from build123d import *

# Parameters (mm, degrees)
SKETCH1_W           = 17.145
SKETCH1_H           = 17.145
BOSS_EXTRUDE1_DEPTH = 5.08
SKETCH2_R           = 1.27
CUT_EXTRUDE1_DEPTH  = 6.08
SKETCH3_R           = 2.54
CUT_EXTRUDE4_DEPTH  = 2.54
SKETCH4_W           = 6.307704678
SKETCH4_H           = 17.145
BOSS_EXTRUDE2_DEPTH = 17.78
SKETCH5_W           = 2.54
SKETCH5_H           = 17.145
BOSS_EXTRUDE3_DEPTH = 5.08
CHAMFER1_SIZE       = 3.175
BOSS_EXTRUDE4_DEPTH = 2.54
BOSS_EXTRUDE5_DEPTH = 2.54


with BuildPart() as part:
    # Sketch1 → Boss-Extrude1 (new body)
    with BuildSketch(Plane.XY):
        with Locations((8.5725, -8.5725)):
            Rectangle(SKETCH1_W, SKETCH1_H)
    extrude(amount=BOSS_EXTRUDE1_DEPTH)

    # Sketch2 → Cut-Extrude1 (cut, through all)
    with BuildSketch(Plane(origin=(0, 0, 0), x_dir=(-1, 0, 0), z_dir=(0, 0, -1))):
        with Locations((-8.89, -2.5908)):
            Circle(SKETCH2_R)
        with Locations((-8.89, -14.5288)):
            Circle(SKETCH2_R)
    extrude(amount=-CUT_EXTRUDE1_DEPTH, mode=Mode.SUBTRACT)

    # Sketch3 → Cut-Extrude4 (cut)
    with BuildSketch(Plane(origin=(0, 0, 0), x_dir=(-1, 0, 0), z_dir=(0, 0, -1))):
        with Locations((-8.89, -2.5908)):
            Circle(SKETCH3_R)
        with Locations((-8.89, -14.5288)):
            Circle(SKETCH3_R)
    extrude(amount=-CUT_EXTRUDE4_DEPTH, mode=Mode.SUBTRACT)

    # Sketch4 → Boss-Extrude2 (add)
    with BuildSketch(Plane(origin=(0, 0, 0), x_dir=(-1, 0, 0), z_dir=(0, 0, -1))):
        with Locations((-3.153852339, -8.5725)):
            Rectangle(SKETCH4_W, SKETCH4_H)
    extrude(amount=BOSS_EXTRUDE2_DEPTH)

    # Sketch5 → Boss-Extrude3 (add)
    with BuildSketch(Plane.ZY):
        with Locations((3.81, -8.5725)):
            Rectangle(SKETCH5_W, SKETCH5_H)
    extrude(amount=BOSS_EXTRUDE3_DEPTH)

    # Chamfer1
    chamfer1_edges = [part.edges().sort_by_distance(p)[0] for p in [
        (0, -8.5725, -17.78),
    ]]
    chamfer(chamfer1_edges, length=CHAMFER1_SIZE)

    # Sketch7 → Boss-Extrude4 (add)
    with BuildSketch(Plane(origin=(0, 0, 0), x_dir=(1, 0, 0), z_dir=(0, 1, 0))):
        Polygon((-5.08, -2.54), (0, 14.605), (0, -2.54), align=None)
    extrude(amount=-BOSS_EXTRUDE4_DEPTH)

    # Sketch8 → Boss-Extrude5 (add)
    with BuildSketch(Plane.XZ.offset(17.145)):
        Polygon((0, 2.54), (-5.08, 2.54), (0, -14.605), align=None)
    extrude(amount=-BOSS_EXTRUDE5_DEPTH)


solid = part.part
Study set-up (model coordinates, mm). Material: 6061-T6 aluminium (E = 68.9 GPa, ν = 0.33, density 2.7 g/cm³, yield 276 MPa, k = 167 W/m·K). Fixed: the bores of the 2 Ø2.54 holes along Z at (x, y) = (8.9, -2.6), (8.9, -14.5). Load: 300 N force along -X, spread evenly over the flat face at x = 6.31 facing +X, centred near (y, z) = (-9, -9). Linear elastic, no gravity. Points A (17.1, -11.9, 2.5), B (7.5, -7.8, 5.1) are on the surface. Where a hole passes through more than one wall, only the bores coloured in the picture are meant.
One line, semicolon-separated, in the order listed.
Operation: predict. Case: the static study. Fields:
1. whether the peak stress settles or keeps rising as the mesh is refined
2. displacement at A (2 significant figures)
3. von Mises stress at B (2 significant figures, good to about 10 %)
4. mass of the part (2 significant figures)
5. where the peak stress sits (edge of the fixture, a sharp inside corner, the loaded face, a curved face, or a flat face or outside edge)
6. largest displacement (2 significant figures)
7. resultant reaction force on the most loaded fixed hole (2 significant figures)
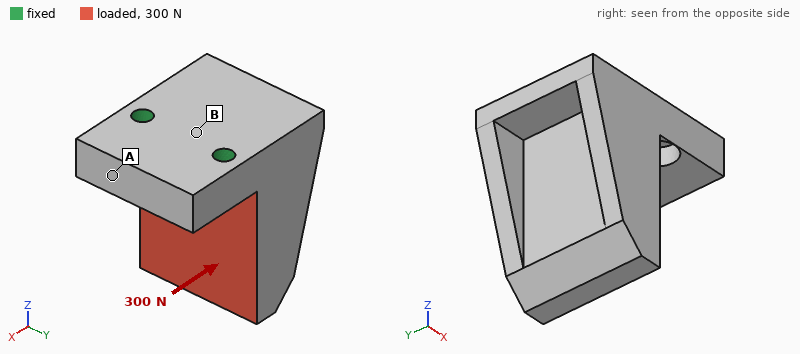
keeps rising; 16 µm; 40 MPa; 9.8 g; edge of the fixture; 88 µm; 150 N
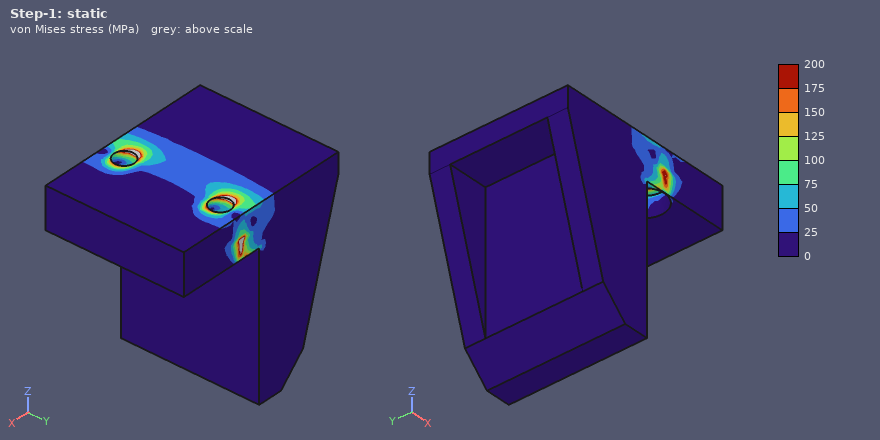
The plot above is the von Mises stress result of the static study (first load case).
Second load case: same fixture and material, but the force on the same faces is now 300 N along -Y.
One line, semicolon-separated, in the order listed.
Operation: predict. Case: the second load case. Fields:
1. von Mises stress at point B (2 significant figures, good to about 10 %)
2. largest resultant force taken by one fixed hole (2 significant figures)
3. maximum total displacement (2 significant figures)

8.2 MPa; 340 N; 19 µm
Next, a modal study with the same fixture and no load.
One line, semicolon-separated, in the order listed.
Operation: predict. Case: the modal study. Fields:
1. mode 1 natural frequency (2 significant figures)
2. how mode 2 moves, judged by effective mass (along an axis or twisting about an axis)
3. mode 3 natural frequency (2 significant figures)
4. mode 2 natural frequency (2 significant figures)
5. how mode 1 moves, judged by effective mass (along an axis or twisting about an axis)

4600 Hz; along Y; 21 kHz; 11 kHz; along X
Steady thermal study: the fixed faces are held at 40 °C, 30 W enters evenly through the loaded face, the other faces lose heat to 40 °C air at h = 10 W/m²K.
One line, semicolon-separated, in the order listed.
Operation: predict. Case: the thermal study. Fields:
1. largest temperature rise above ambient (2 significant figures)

32 K
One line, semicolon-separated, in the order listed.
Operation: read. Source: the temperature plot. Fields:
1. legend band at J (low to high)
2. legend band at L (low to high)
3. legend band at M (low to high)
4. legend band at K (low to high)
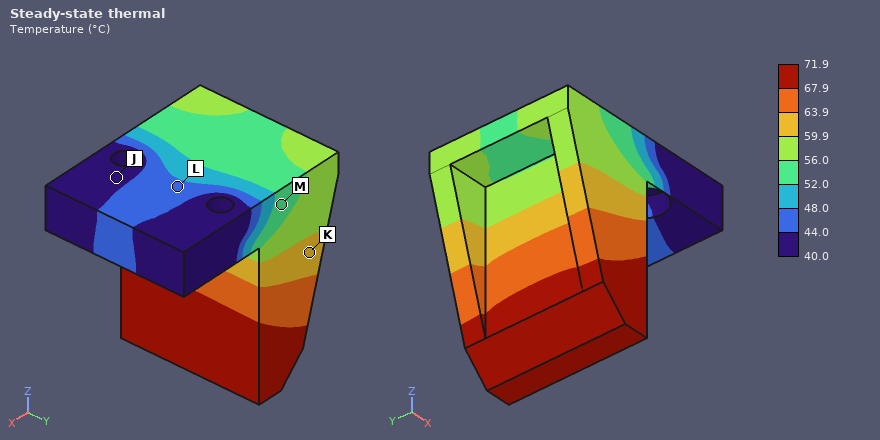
40.0 to 44.0 °C; 44.0 to 48.0 °C; 52.0 to 56.0 °C; 59.9 to 63.9 °C
